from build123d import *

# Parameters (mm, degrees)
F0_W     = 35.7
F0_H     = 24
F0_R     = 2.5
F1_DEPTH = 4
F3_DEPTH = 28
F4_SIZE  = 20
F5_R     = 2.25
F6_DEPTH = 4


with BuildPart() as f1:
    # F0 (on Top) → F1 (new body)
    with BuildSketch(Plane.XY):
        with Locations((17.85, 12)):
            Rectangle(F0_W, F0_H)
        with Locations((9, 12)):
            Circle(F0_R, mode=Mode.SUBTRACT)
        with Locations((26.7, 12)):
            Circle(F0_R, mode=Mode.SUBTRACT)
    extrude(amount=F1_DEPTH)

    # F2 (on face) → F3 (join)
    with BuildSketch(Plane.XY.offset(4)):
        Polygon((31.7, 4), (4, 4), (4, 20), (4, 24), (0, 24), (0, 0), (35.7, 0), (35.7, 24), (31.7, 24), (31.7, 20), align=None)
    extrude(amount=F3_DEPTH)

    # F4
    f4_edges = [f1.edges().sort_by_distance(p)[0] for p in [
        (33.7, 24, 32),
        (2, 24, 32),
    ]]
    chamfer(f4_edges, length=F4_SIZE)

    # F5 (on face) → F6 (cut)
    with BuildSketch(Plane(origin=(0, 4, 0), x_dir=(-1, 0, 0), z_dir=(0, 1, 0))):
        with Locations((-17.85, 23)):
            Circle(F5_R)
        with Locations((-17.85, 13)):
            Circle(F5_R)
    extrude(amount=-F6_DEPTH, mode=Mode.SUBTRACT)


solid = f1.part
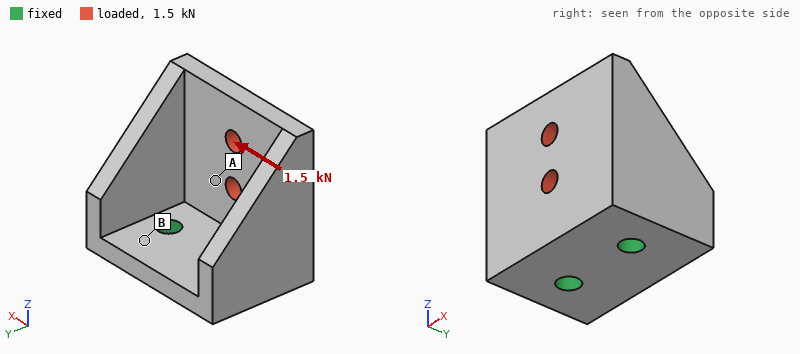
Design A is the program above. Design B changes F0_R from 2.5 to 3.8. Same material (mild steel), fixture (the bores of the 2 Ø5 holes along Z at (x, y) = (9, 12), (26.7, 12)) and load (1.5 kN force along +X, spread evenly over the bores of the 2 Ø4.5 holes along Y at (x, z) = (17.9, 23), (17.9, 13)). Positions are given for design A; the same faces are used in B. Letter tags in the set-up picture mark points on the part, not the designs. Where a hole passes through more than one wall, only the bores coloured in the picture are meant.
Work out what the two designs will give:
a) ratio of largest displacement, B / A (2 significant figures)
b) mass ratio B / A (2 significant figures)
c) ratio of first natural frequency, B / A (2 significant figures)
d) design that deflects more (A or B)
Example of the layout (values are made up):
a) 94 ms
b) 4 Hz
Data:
a) 0.71
b) 0.98
c) 1.3
d) A
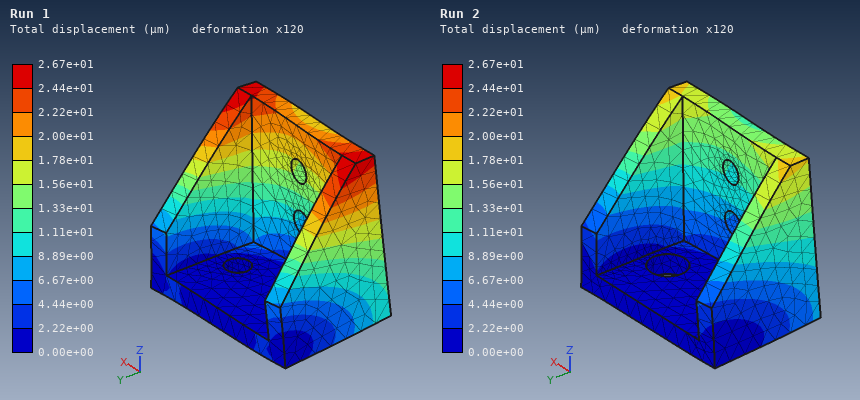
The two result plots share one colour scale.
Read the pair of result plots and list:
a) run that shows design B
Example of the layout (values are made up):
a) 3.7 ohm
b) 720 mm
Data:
a) Run 2
